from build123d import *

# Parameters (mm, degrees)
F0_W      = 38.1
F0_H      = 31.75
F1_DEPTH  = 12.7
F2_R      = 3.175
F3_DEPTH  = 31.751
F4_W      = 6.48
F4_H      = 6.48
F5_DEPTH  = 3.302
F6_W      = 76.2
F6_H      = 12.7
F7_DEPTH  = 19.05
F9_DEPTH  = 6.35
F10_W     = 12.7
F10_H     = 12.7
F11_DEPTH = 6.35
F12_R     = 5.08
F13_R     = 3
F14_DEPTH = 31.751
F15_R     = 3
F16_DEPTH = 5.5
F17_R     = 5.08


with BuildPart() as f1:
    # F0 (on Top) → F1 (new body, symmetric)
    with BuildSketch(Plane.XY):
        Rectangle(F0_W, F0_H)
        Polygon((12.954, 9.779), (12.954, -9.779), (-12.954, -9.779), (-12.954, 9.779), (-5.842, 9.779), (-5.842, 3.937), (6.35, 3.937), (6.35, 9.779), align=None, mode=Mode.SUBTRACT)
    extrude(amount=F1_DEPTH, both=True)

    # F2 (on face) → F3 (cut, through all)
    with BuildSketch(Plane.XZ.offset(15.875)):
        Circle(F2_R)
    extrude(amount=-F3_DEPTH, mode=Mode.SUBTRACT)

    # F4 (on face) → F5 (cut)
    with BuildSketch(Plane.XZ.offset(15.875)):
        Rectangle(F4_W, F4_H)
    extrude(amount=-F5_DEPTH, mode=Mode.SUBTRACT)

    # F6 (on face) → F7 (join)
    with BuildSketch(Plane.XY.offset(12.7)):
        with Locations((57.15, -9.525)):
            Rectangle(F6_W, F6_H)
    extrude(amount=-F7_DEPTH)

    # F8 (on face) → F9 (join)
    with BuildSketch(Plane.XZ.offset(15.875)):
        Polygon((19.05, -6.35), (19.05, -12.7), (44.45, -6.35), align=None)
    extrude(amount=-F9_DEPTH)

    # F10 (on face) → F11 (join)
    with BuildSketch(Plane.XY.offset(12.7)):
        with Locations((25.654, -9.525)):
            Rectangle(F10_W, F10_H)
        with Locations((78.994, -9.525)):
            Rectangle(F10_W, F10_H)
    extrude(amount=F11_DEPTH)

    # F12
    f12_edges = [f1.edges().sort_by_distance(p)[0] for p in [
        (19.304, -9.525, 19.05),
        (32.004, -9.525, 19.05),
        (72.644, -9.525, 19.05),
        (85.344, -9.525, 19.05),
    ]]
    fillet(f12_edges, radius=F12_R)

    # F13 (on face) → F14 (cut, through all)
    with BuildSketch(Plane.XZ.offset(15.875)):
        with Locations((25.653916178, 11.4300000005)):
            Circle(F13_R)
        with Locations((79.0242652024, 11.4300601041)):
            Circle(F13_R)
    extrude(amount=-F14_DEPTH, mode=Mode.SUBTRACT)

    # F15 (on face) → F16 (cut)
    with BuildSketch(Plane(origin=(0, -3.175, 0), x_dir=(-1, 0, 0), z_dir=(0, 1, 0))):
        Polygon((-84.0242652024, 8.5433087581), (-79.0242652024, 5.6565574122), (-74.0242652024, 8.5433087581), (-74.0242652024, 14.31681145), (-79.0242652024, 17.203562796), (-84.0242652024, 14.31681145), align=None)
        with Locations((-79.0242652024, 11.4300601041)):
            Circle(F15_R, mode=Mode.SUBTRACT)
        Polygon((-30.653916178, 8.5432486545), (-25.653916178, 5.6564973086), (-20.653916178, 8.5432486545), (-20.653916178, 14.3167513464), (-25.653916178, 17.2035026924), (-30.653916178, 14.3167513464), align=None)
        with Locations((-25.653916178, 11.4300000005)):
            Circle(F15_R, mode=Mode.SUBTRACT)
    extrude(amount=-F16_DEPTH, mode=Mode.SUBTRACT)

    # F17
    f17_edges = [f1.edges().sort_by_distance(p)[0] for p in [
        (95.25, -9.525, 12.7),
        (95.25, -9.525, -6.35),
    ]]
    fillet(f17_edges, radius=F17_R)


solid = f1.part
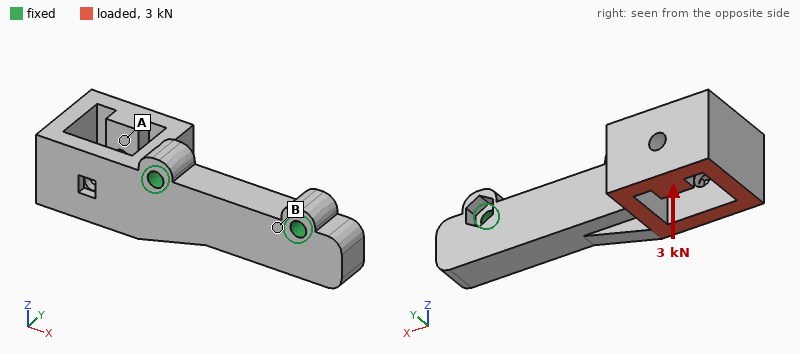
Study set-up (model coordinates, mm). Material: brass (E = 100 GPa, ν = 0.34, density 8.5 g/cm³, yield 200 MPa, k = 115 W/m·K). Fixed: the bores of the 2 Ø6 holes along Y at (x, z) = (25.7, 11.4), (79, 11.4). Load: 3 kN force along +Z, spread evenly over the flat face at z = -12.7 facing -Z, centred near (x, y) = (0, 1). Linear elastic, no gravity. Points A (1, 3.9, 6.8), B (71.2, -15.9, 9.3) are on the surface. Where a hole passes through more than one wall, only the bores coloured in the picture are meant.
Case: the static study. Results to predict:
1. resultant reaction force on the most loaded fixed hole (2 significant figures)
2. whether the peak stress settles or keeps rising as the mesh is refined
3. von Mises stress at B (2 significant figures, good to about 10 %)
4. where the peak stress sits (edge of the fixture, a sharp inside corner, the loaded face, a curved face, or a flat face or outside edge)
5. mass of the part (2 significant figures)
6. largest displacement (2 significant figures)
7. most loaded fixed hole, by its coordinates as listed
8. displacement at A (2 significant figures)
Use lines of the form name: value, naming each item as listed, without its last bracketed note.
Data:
resultant reaction force on the most loaded fixed hole: 4.5 kN
whether the peak stress settles or keeps rising as the mesh is refined: keeps rising
von Mises stress at B: 39 MPa
where the peak stress sits: a sharp inside corner
mass of the part: 330 g
largest displacement: 0.21 mm
most loaded fixed hole, by its coordinates as listed: (25.7, 11.4)
displacement at A: 0.098 mm
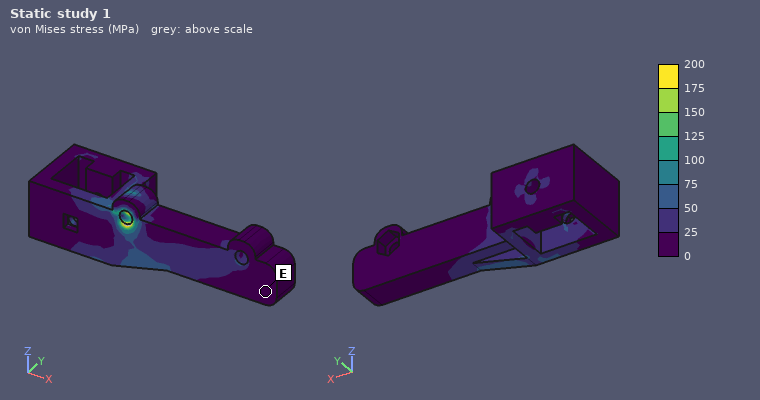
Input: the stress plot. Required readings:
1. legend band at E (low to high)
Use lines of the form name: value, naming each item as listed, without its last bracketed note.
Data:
legend band at E: 0 to 25 MPa
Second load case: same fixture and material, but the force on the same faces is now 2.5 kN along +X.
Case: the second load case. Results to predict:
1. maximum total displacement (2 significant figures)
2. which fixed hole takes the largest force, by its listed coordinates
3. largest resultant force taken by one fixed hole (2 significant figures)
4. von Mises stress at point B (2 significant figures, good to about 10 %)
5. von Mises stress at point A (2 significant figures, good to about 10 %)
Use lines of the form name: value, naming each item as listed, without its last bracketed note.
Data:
maximum total displacement: 0.15 mm
which fixed hole takes the largest force, by its listed coordinates: (79, 11.4)
largest resultant force taken by one fixed hole: 2.4 kN
von Mises stress at point B: 27 MPa
von Mises stress at point A: 12 MPa
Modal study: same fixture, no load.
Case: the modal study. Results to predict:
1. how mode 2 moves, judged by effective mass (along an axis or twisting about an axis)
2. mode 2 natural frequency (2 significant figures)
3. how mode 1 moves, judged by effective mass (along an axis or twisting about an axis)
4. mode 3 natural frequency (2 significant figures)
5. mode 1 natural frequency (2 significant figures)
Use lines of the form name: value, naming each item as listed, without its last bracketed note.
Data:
how mode 2 moves, judged by effective mass: along Z
mode 2 natural frequency: 1900 Hz
how mode 1 moves, judged by effective mass: along Y
mode 3 natural frequency: 3700 Hz
mode 1 natural frequency: 1300 Hz
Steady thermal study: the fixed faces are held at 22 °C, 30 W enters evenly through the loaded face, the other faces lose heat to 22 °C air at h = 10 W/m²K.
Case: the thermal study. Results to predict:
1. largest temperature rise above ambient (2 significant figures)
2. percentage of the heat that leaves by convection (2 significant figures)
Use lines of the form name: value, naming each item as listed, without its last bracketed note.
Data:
largest temperature rise above ambient: 37 K
percentage of the heat that leaves by convection: 7.1 %
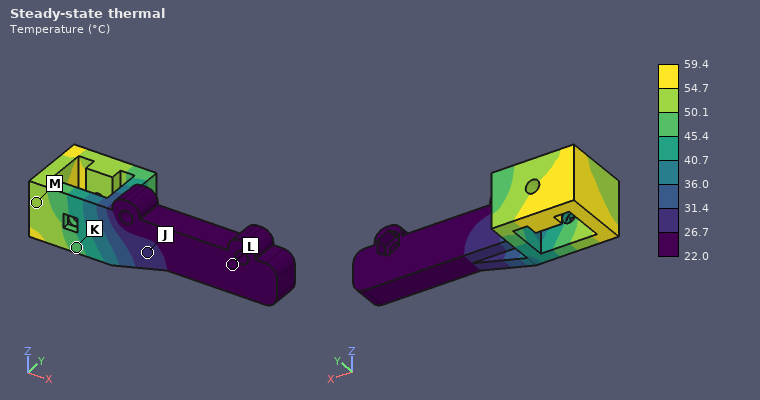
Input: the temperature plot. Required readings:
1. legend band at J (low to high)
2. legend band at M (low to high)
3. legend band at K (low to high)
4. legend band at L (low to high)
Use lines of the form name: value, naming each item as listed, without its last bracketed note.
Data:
legend band at J: 26.7 to 31.4 °C
legend band at M: 50.1 to 54.7 °C
legend band at K: 45.4 to 50.1 °C
legend band at L: 22.0 to 26.7 °C
